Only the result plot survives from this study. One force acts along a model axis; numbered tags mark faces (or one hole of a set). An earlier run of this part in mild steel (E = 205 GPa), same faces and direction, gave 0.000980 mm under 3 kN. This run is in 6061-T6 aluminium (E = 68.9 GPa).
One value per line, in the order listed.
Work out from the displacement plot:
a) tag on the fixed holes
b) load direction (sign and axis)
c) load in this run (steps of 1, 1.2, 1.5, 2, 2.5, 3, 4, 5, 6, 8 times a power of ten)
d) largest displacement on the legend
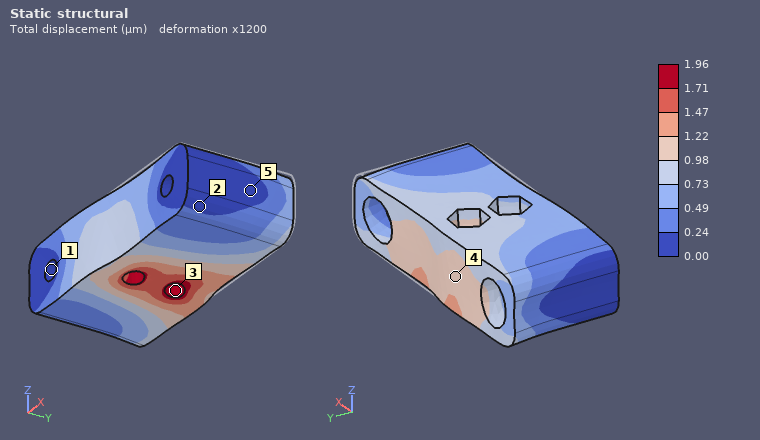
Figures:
1
-X
2 kN
1.96 µm
